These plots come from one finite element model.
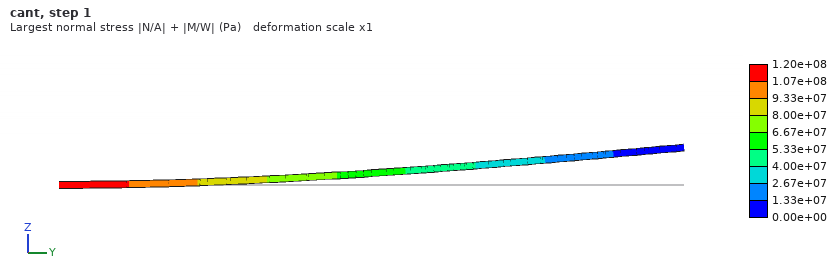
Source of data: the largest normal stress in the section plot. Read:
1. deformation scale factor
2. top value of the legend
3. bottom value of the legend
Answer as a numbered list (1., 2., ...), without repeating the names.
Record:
1. 1
2. 1.20e+08 Pa
3. 0.00e+00 Pa
